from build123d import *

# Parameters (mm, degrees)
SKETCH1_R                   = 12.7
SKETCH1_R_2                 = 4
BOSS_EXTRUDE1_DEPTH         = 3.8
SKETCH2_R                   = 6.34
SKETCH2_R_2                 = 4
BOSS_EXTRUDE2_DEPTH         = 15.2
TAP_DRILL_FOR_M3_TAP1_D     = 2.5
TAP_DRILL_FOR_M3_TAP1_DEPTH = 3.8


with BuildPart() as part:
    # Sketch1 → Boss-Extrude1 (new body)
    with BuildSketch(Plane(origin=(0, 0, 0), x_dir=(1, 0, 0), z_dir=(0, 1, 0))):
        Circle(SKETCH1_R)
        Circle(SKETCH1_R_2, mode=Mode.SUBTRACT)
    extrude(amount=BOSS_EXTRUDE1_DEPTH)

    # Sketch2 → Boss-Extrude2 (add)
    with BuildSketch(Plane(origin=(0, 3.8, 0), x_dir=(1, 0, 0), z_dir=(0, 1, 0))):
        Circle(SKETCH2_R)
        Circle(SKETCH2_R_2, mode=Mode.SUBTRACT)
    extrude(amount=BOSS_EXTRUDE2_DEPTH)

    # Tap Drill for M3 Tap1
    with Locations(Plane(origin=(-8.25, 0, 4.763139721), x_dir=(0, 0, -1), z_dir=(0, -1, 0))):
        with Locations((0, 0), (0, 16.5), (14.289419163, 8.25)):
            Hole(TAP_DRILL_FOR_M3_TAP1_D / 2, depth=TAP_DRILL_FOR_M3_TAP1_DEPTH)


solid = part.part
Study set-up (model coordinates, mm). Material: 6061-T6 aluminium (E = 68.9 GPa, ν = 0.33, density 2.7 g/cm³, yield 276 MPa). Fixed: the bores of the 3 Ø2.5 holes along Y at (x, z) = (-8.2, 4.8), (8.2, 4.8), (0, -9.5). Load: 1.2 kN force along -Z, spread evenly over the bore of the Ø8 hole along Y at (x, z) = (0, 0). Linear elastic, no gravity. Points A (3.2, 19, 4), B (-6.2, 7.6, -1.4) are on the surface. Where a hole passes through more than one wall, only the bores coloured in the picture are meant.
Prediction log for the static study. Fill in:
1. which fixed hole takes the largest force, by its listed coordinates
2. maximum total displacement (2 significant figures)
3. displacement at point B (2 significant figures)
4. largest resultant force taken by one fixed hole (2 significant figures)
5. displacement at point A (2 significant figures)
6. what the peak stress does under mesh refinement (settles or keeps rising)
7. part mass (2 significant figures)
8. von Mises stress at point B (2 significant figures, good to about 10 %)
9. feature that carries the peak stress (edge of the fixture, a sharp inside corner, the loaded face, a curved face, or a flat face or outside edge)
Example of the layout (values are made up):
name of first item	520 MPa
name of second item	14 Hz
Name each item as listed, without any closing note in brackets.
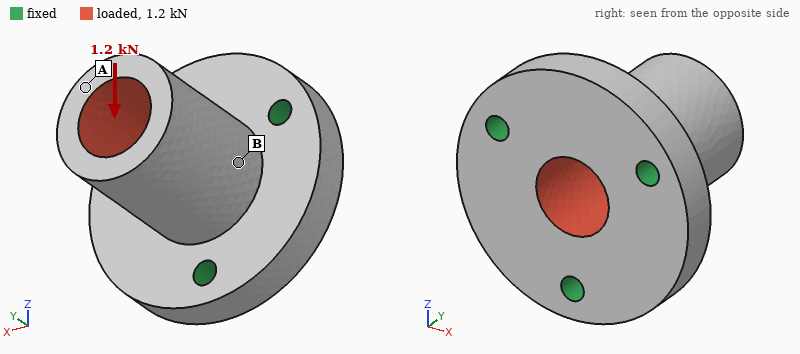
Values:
which fixed hole takes the largest force, by its listed coordinates	(0, -9.5)
maximum total displacement	28 µm
displacement at point B	8.3 µm
largest resultant force taken by one fixed hole	760 N
displacement at point A	27 µm
what the peak stress does under mesh refinement	keeps rising
part mass	7.7 g
von Mises stress at point B	23 MPa
feature that carries the peak stress	edge of the fixture
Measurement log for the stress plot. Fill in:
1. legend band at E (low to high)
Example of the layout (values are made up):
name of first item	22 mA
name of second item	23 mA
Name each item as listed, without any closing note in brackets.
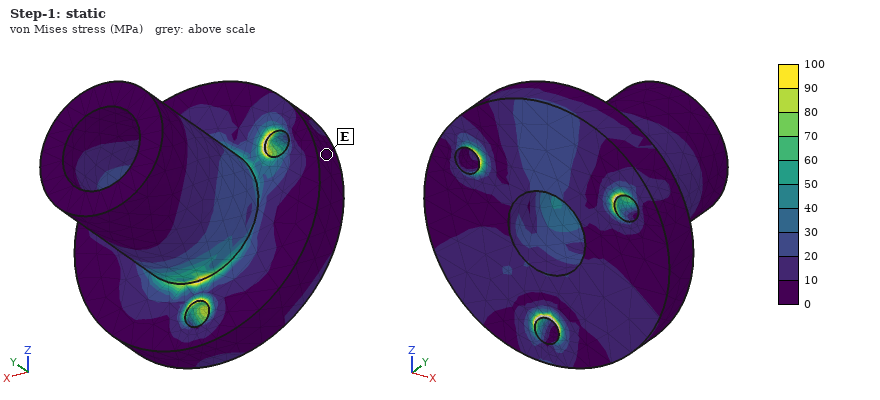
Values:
legend band at E	0 to 10 MPa
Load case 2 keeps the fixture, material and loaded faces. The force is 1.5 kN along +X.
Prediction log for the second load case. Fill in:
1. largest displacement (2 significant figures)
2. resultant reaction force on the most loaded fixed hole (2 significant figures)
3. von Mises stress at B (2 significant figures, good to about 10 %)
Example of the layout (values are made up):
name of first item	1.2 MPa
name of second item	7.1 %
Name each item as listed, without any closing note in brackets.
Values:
largest displacement	35 µm
resultant reaction force on the most loaded fixed hole	860 N
von Mises stress at B	25 MPa
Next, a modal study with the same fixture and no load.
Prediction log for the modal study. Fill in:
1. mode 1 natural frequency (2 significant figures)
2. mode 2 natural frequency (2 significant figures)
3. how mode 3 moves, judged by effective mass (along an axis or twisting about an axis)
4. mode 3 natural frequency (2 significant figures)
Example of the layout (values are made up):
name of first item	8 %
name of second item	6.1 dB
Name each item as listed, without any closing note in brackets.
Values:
mode 1 natural frequency	19 kHz
mode 2 natural frequency	19 kHz
how mode 3 moves, judged by effective mass	along Y
mode 3 natural frequency	37 kHz
